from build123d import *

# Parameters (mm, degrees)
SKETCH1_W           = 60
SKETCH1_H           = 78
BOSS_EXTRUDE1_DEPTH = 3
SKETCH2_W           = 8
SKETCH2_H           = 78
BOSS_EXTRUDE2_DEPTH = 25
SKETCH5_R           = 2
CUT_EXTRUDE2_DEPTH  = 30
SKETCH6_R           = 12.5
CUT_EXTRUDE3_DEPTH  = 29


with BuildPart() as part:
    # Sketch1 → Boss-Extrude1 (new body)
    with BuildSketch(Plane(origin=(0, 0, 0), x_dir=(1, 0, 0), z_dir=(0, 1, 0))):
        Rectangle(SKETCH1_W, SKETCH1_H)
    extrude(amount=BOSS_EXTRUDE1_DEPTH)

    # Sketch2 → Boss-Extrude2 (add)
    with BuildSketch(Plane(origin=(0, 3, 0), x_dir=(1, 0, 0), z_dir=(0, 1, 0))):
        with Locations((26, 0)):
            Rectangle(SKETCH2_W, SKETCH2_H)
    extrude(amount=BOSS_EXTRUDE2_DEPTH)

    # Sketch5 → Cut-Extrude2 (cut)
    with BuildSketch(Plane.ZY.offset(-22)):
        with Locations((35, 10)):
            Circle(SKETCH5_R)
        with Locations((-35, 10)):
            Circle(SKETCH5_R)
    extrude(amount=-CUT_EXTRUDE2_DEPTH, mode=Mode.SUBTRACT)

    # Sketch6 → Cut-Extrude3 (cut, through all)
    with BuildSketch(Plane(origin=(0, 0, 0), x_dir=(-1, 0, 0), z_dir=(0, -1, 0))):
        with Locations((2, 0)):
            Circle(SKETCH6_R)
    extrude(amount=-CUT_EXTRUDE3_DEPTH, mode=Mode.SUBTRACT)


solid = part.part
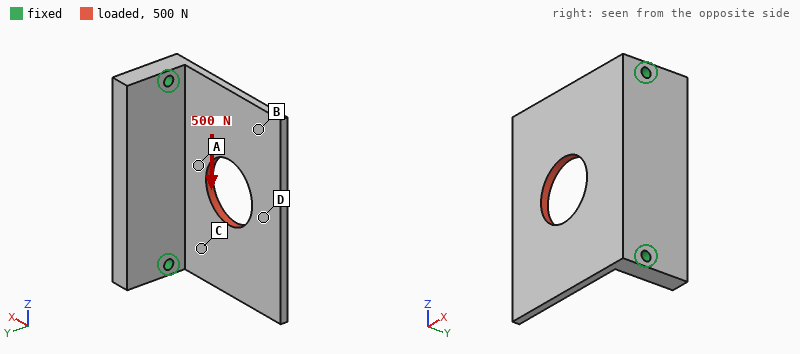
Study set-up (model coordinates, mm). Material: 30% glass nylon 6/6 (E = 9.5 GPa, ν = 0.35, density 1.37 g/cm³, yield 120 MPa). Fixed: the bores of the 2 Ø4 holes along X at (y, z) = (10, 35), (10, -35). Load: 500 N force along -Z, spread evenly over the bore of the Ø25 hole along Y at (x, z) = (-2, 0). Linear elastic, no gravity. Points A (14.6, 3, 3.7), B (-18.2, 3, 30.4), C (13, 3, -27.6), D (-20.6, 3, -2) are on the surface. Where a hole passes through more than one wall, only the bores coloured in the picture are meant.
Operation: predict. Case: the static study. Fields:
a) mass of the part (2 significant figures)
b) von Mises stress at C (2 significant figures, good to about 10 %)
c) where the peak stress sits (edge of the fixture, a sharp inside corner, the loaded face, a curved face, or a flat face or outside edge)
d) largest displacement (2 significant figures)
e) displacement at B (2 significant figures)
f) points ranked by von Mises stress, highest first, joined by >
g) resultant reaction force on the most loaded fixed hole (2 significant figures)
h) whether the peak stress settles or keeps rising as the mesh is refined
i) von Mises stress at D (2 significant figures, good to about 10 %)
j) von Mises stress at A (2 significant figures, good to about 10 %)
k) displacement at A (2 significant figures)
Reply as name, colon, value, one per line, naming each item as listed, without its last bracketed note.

mass of the part: 38 g
von Mises stress at C: 4.5 MPa
where the peak stress sits: edge of the fixture
largest displacement: 79 µm
displacement at B: 64 µm
points ranked by von Mises stress, highest first, joined by >: A > C > D > B
resultant reaction force on the most loaded fixed hole: 330 N
whether the peak stress settles or keeps rising as the mesh is refined: keeps rising
von Mises stress at D: 2.7 MPa
von Mises stress at A: 6.7 MPa
displacement at A: 15 µm
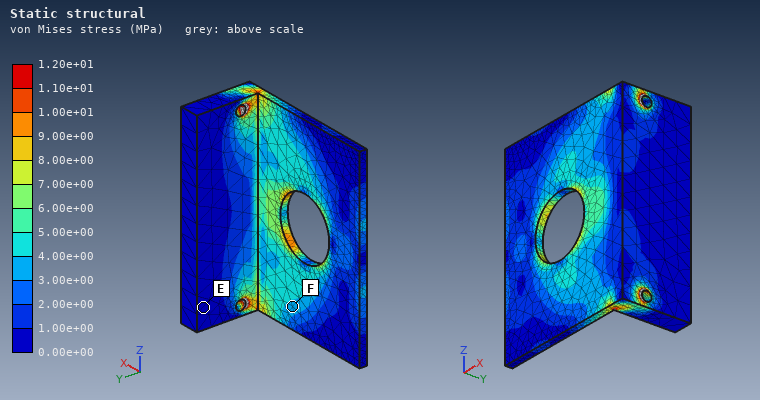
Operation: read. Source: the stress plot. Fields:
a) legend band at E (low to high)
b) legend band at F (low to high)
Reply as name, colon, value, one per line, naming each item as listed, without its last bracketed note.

legend band at E: 0.00e+00 to 1.00e+00 MPa
legend band at F: 3.00e+00 to 4.00e+00 MPa
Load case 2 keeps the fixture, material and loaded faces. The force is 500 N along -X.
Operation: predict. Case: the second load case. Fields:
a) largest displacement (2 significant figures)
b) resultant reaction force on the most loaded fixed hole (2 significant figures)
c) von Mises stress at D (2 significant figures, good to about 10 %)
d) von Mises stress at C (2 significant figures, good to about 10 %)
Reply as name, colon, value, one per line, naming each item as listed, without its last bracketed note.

largest displacement: 0.12 mm
resultant reaction force on the most loaded fixed hole: 260 N
von Mises stress at D: 2.7 MPa
von Mises stress at C: 3.6 MPa
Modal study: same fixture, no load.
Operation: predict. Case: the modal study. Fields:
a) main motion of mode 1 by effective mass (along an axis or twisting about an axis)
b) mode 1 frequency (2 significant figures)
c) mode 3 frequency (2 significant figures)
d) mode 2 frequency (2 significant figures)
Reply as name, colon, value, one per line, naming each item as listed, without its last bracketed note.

main motion of mode 1 by effective mass: along Y
mode 1 frequency: 420 Hz
mode 3 frequency: 1800 Hz
mode 2 frequency: 770 Hz
